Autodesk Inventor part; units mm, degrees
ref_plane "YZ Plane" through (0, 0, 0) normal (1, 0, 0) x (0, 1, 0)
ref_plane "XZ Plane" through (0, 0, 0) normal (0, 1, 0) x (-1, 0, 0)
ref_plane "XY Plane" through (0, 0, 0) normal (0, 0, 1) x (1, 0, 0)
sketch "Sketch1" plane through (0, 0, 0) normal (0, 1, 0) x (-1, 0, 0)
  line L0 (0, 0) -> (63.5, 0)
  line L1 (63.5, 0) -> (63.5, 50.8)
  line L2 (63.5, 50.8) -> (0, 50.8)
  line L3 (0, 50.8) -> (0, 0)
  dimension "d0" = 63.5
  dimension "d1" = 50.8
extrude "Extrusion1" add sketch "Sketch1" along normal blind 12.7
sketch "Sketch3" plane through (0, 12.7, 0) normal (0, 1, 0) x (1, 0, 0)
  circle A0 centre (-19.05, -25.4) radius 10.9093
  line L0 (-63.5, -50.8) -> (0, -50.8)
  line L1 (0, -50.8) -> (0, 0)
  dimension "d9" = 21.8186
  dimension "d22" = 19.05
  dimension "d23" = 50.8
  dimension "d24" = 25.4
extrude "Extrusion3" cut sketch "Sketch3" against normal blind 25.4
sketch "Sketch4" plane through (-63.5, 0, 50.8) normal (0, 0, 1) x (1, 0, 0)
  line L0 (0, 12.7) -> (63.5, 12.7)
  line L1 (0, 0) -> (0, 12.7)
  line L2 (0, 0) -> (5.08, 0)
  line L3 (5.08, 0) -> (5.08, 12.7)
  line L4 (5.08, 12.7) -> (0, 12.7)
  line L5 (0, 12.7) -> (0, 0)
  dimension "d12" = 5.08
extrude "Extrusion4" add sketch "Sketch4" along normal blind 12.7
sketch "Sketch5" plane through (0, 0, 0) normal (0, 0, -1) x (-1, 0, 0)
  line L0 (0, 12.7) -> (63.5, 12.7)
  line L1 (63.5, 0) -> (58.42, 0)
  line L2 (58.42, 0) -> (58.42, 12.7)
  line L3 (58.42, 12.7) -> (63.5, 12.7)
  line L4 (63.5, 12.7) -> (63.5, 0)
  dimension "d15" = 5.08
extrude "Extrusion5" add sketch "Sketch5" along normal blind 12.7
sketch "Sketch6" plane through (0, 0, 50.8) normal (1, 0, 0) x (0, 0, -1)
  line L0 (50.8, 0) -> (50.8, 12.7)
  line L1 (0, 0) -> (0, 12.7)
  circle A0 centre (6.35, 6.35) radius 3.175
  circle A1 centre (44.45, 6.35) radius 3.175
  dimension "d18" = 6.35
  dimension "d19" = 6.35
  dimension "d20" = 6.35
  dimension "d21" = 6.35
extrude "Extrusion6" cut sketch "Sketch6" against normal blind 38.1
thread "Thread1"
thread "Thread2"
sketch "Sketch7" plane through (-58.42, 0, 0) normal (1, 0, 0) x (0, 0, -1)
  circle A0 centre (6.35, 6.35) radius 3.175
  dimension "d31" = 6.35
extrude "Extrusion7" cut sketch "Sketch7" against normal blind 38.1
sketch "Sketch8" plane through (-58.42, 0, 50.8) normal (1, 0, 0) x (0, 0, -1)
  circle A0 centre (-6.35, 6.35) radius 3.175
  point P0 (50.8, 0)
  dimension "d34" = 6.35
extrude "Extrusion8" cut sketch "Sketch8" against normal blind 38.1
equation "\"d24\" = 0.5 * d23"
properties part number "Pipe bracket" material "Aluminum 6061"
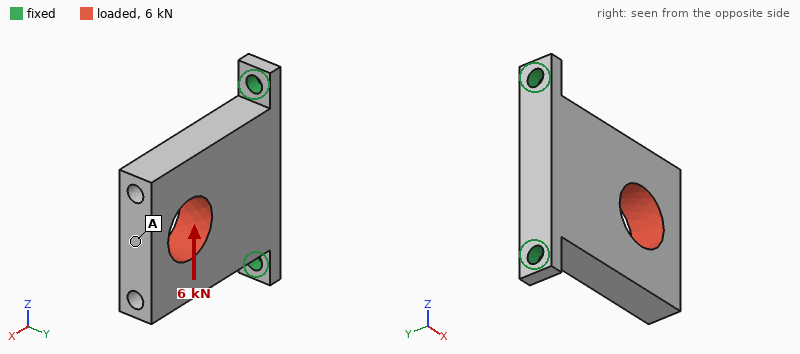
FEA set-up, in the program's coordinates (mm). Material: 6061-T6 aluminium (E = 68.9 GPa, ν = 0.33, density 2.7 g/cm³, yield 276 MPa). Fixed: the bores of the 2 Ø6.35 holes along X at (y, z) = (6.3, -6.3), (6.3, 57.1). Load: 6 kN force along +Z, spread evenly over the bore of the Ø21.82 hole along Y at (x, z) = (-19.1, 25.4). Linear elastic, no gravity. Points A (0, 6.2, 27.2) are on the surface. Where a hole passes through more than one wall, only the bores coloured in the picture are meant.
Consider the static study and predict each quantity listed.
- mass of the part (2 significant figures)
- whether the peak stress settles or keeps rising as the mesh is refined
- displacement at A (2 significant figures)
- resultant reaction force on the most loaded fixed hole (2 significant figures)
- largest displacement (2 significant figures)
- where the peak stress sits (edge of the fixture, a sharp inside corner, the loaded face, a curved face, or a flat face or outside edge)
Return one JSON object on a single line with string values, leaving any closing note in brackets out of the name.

{"mass of the part": "95 g", "whether the peak stress settles or keeps rising as the mesh is refined": "keeps rising", "displacement at A": "0.13 mm", "resultant reaction force on the most loaded fixed hole": "5.6 kN", "largest displacement": "0.15 mm", "where the peak stress sits": "edge of the fixture"}
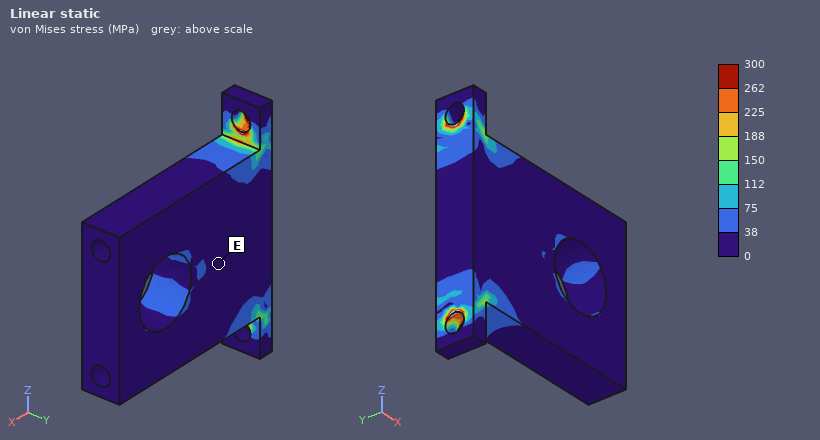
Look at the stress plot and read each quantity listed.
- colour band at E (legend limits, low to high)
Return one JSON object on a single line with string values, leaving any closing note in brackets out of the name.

{"colour band at E": "0 to 38 MPa"}
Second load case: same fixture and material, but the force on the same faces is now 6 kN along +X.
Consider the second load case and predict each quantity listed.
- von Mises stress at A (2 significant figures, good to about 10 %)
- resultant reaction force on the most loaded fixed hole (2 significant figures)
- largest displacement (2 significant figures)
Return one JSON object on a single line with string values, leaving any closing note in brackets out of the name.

{"von Mises stress at A": "21 MPa", "resultant reaction force on the most loaded fixed hole": "3.4 kN", "largest displacement": "39 µm"}
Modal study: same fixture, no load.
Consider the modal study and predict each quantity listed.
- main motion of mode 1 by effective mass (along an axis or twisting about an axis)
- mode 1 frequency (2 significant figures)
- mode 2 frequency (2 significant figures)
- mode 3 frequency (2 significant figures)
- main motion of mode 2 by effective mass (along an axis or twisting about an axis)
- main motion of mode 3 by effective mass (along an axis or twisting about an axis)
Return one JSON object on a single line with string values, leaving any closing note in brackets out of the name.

{"main motion of mode 1 by effective mass": "along Y", "mode 1 frequency": "1000 Hz", "mode 2 frequency": "5200 Hz", "mode 3 frequency": "5600 Hz", "main motion of mode 2 by effective mass": "along Z", "main motion of mode 3 by effective mass": "twisting about X"}
